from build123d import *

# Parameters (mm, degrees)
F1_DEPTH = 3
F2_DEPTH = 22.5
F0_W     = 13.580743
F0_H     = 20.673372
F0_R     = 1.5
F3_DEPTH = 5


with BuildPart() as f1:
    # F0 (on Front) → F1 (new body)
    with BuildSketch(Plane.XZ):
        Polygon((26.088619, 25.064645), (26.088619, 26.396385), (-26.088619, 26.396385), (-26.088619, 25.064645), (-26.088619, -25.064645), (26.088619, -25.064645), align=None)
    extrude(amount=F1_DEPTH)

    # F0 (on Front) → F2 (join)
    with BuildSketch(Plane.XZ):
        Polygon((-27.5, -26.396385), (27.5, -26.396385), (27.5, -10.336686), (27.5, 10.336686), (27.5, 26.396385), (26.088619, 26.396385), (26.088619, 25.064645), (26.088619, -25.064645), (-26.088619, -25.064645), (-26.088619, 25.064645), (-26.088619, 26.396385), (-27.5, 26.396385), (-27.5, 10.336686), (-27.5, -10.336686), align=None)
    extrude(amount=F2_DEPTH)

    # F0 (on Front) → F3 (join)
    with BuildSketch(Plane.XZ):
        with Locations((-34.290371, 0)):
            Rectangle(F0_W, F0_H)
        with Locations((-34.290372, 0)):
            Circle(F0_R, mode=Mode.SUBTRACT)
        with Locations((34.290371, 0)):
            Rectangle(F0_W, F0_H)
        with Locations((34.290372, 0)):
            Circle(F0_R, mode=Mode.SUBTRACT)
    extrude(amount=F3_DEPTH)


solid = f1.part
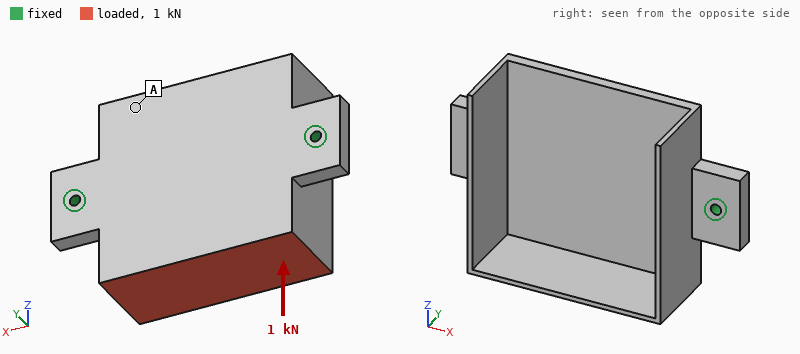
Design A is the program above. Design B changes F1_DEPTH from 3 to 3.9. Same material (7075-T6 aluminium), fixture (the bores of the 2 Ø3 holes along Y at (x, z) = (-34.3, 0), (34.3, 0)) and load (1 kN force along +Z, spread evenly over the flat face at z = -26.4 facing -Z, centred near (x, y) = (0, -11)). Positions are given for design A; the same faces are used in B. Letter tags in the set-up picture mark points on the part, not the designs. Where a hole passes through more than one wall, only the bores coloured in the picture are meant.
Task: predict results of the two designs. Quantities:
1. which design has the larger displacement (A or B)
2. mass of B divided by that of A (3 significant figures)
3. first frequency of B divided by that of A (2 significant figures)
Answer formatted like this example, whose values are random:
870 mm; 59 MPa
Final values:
A; 1.15; 1.00
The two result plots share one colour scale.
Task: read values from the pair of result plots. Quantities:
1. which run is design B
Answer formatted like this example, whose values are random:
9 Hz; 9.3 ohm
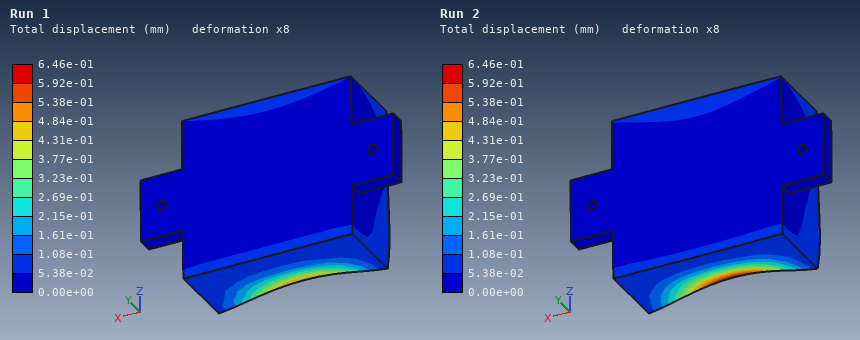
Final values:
Run 1
